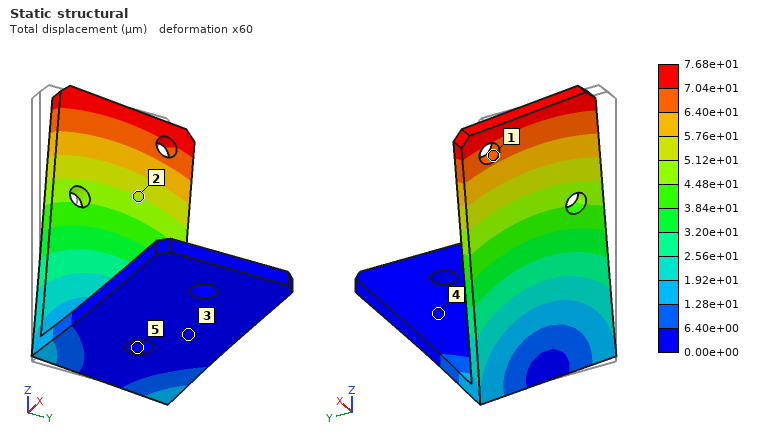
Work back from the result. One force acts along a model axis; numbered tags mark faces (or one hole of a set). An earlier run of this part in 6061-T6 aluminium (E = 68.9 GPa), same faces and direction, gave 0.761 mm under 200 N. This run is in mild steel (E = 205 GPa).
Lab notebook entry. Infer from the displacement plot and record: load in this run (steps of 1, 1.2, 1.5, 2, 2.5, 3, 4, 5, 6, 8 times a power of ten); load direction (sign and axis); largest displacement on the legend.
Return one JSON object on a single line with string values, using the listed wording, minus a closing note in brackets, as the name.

{"load in this run": "60 N", "load direction": "+Y", "largest displacement on the legend": "7.68e+01 µm"}
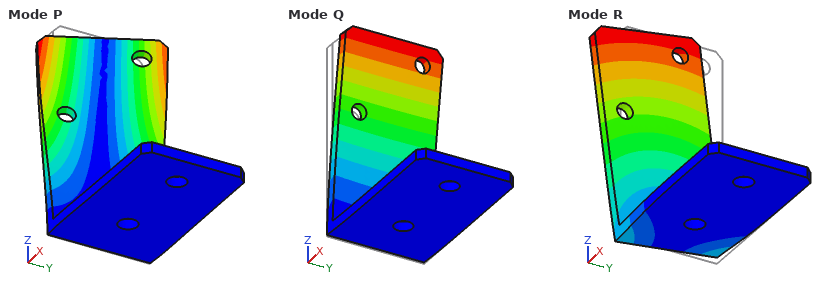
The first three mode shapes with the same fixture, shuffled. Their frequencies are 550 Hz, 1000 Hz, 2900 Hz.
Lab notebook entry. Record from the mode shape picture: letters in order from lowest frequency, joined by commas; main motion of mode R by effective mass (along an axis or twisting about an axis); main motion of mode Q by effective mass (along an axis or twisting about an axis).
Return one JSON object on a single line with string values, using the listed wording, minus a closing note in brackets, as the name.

{"letters in order from lowest frequency, joined by commas": "Q, R, P", "main motion of mode R by effective mass": "along Y", "main motion of mode Q by effective mass": "along X"}
